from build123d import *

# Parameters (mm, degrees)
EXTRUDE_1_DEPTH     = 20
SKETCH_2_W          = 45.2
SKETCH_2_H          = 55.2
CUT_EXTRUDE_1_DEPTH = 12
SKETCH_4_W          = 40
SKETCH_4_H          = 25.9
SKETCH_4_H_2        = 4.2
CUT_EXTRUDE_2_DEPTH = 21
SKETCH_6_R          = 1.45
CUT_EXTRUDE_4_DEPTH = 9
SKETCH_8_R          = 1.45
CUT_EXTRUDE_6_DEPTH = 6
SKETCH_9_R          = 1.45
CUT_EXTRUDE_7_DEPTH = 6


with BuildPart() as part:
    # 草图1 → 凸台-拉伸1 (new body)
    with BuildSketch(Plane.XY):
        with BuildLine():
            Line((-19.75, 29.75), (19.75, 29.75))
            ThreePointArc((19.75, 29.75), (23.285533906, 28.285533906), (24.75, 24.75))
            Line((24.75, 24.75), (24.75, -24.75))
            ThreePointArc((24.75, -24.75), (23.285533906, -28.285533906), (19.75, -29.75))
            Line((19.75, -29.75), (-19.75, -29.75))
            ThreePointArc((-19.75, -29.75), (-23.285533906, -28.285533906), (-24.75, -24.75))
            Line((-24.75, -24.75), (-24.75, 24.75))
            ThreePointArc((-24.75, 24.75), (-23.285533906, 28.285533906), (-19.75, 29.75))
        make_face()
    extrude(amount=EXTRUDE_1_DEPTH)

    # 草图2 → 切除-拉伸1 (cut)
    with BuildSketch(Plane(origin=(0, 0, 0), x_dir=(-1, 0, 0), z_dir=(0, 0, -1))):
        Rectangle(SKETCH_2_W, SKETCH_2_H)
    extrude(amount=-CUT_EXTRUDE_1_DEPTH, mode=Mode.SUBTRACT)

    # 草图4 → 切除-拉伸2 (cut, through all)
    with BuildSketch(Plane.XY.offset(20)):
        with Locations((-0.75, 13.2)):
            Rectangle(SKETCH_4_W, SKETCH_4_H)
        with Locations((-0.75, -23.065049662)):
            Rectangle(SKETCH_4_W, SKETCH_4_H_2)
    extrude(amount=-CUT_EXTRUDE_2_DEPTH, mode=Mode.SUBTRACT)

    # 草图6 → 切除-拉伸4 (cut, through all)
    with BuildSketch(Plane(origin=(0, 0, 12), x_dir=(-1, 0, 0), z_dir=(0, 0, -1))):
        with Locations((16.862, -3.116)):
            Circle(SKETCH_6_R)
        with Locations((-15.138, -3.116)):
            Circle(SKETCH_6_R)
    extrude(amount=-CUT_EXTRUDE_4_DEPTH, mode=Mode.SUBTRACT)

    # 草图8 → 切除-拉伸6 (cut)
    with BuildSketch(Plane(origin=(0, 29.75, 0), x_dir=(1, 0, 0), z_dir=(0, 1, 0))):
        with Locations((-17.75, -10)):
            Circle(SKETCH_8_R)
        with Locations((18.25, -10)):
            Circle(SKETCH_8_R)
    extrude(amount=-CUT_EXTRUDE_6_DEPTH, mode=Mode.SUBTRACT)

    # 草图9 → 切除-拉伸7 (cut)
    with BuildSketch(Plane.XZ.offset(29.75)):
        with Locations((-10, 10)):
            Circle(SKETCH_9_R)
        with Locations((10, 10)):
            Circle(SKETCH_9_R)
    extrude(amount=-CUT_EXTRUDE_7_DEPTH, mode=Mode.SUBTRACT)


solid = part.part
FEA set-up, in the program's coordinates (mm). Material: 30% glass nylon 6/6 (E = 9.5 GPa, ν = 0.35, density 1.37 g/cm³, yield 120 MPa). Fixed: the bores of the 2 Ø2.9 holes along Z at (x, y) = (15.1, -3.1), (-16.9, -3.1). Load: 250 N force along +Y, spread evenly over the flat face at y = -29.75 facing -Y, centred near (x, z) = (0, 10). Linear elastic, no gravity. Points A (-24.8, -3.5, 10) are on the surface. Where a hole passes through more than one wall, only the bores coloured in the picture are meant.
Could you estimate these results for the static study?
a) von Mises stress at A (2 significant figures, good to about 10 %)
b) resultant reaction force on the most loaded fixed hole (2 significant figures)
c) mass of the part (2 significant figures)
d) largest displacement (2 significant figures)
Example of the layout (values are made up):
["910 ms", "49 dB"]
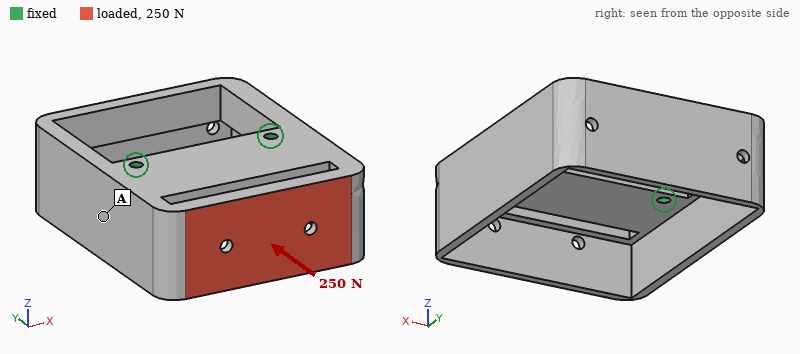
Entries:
["3.2 MPa", "140 N", "26 g", "0.39 mm"]
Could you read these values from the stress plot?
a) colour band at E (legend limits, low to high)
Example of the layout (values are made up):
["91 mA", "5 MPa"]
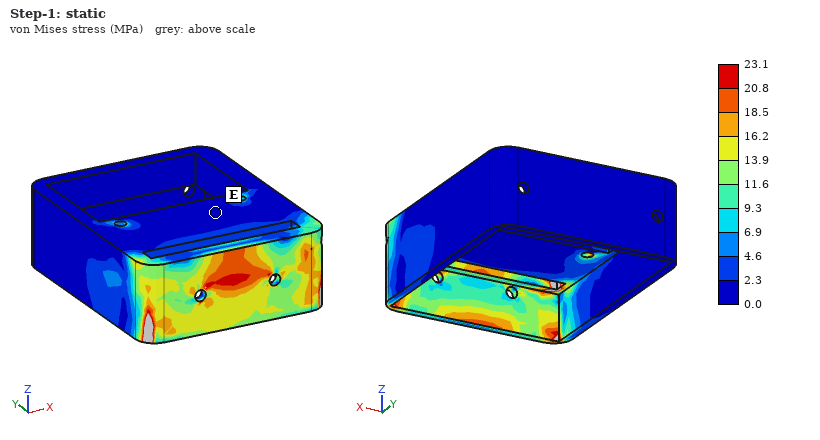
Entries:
["0.0 to 2.3 MPa"]
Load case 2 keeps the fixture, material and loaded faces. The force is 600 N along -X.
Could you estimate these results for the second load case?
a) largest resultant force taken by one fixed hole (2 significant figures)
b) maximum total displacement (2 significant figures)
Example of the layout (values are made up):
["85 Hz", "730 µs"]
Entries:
["570 N", "0.18 mm"]
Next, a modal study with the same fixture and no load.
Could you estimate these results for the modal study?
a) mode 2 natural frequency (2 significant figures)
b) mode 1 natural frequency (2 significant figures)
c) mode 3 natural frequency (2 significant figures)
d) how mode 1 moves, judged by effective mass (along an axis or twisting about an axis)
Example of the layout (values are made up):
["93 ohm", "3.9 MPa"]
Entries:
["1800 Hz", "1300 Hz", "2700 Hz", "along X"]
